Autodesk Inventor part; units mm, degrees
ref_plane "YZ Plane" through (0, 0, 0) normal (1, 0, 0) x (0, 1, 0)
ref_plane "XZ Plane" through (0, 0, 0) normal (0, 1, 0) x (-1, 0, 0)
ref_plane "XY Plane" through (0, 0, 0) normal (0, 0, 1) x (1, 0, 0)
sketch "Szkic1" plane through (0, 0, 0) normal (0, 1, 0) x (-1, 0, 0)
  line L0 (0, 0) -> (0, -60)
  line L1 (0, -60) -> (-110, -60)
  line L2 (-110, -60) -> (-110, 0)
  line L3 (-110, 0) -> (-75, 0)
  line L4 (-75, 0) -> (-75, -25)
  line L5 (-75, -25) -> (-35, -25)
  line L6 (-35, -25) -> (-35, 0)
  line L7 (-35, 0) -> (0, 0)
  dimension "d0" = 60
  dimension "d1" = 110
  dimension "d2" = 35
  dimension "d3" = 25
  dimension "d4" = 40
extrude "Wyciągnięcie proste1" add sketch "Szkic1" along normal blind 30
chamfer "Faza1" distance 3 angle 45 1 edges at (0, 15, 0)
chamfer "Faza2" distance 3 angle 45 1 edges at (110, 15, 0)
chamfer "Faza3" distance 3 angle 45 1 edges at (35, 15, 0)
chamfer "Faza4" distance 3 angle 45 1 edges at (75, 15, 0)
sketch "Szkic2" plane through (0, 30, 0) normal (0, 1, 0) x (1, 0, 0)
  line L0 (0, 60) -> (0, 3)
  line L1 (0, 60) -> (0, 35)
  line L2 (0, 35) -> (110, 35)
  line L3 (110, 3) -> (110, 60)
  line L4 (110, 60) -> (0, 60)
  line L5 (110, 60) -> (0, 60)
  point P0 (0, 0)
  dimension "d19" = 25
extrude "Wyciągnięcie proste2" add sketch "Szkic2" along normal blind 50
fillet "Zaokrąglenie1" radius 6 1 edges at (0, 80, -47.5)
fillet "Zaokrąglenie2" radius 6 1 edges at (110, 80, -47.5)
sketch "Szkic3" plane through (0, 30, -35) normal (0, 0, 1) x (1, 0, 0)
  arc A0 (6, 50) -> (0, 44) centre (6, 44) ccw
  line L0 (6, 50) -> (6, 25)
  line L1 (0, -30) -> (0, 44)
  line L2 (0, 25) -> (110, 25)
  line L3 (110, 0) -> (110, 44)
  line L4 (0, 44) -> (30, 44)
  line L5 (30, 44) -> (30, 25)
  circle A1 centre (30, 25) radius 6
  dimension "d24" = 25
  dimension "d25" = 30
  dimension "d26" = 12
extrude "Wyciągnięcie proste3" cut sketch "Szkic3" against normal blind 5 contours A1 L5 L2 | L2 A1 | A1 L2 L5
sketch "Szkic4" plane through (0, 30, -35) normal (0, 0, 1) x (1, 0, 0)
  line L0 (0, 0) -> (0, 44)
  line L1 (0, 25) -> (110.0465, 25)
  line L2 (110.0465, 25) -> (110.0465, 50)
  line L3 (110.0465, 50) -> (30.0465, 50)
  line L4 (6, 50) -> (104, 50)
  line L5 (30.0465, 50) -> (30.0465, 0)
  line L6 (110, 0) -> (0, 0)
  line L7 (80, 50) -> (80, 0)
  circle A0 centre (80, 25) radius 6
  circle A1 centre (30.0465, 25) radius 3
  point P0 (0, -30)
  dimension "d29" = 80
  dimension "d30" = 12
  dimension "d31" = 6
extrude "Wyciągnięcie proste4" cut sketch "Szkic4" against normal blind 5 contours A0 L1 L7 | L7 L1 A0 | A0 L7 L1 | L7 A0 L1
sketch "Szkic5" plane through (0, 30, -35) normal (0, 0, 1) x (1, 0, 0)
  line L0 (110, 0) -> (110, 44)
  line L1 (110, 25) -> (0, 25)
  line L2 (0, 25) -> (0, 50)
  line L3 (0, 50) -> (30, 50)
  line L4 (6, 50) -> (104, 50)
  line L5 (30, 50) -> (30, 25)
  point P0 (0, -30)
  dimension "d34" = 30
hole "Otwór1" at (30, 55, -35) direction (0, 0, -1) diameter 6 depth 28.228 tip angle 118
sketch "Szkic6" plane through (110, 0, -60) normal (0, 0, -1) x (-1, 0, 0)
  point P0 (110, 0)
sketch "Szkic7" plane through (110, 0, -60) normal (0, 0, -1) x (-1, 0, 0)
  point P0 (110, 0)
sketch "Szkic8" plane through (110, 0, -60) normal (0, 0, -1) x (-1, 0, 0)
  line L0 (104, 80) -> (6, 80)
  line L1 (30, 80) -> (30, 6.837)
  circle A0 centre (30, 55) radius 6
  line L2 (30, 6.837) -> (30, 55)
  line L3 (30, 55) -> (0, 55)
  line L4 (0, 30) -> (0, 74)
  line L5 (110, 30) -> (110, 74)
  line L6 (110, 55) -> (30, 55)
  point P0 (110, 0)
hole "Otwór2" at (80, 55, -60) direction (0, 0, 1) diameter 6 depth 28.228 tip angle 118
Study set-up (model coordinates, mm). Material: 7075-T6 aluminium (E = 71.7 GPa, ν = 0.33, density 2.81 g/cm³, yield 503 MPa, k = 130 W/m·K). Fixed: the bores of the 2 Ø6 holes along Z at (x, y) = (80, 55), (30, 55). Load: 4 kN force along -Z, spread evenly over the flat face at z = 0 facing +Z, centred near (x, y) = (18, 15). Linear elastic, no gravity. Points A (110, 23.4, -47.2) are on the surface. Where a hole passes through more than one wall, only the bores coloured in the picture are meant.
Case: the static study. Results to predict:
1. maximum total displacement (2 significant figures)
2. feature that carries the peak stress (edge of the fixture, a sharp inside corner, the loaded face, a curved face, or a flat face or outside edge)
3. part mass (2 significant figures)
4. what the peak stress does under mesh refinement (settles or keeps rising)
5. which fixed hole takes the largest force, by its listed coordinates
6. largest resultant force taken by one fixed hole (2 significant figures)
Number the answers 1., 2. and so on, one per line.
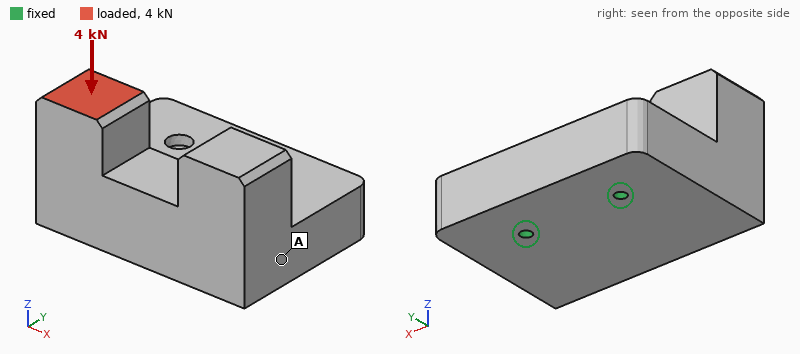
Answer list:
1. 73 µm
2. edge of the fixture
3. 850 g
4. keeps rising
5. (30, 55)
6. 4.3 kN
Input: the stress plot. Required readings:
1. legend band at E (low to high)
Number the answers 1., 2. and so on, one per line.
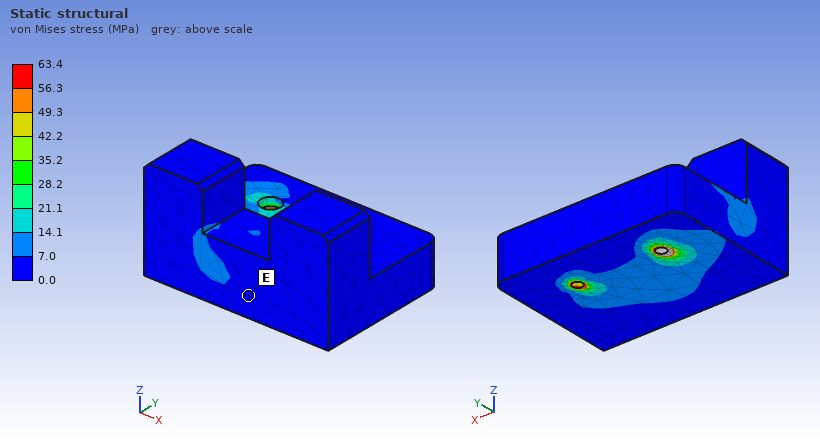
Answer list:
1. 0.0 to 7.0 MPa
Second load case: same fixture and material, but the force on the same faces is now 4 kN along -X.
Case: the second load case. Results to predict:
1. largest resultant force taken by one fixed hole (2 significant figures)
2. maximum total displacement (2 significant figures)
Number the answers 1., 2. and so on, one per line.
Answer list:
1. 4.9 kN
2. 55 µm
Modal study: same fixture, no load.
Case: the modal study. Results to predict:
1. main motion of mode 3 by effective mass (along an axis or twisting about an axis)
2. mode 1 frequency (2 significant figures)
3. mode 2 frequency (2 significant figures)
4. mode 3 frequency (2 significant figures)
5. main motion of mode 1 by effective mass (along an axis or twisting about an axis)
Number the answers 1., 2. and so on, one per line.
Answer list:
1. along X
2. 2300 Hz
3. 3800 Hz
4. 5100 Hz
5. along Z
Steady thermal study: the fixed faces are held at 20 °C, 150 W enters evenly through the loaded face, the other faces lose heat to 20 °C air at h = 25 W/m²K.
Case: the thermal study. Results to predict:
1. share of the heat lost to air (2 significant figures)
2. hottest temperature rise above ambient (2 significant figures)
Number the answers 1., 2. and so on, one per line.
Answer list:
1. 9.2 %
2. 69 K
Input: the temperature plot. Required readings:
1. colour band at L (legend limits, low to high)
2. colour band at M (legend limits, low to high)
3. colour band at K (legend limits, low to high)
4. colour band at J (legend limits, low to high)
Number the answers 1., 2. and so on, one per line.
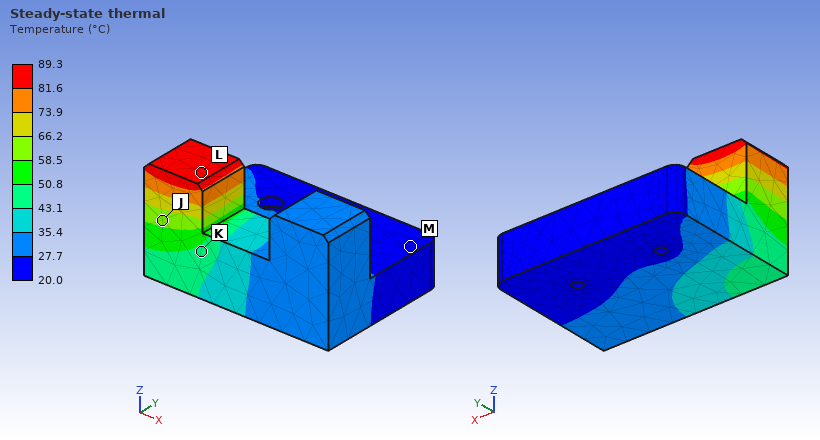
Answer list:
1. 81.6 to 89.3 °C
2. 20.0 to 27.7 °C
3. 43.1 to 50.8 °C
4. 58.5 to 66.2 °C
